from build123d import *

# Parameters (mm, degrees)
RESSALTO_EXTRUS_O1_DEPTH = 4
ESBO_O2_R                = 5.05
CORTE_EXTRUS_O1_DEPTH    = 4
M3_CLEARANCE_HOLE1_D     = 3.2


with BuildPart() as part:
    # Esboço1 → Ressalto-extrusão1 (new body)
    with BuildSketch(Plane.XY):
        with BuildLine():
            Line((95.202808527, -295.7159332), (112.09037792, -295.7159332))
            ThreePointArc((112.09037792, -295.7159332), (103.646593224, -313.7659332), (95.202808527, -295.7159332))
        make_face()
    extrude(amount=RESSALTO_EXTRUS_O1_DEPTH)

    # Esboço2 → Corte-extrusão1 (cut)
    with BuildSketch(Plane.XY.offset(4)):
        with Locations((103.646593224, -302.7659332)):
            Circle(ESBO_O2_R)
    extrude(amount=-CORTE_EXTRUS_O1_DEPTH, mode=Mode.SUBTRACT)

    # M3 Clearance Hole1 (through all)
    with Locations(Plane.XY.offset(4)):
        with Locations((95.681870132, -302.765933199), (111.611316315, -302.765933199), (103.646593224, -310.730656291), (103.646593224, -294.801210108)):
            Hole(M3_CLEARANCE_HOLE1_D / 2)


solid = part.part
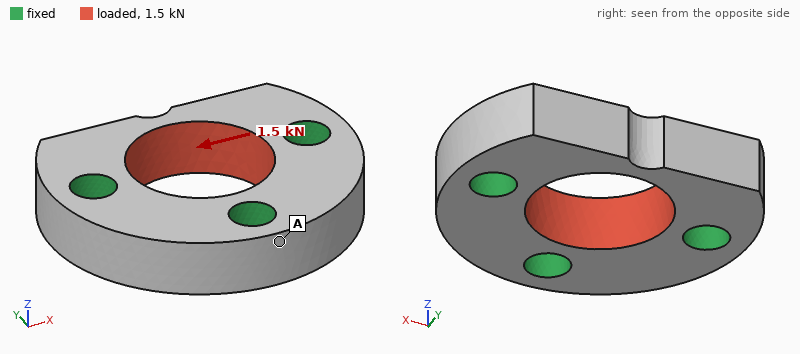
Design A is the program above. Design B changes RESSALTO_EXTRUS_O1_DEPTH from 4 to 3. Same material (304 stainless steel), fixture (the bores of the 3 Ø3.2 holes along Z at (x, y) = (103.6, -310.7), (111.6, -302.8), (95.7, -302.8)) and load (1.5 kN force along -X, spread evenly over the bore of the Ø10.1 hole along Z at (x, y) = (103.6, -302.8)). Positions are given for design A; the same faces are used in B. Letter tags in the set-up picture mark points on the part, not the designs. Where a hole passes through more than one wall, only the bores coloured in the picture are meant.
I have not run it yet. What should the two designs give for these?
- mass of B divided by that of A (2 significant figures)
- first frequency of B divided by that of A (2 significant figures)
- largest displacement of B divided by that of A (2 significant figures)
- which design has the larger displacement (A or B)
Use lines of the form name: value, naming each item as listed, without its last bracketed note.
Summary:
mass of B divided by that of A: 0.75
first frequency of B divided by that of A: 0.82
largest displacement of B divided by that of A: 1.3
which design has the larger displacement: B
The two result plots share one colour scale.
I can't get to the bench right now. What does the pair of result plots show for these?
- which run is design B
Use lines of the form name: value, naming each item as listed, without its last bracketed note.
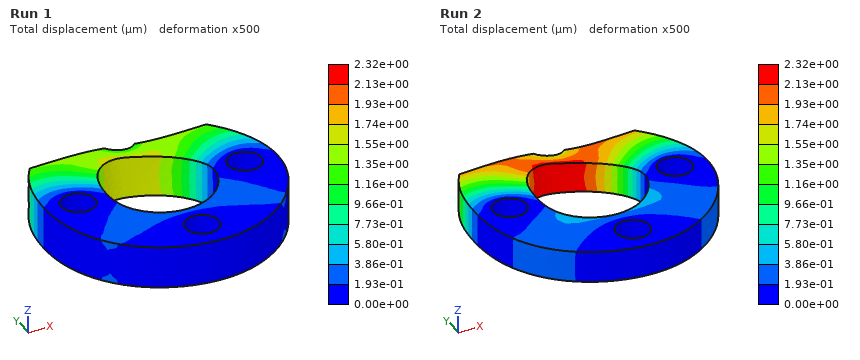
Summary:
which run is design B: Run 2
